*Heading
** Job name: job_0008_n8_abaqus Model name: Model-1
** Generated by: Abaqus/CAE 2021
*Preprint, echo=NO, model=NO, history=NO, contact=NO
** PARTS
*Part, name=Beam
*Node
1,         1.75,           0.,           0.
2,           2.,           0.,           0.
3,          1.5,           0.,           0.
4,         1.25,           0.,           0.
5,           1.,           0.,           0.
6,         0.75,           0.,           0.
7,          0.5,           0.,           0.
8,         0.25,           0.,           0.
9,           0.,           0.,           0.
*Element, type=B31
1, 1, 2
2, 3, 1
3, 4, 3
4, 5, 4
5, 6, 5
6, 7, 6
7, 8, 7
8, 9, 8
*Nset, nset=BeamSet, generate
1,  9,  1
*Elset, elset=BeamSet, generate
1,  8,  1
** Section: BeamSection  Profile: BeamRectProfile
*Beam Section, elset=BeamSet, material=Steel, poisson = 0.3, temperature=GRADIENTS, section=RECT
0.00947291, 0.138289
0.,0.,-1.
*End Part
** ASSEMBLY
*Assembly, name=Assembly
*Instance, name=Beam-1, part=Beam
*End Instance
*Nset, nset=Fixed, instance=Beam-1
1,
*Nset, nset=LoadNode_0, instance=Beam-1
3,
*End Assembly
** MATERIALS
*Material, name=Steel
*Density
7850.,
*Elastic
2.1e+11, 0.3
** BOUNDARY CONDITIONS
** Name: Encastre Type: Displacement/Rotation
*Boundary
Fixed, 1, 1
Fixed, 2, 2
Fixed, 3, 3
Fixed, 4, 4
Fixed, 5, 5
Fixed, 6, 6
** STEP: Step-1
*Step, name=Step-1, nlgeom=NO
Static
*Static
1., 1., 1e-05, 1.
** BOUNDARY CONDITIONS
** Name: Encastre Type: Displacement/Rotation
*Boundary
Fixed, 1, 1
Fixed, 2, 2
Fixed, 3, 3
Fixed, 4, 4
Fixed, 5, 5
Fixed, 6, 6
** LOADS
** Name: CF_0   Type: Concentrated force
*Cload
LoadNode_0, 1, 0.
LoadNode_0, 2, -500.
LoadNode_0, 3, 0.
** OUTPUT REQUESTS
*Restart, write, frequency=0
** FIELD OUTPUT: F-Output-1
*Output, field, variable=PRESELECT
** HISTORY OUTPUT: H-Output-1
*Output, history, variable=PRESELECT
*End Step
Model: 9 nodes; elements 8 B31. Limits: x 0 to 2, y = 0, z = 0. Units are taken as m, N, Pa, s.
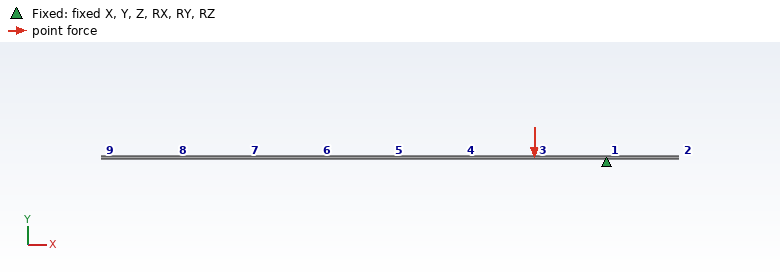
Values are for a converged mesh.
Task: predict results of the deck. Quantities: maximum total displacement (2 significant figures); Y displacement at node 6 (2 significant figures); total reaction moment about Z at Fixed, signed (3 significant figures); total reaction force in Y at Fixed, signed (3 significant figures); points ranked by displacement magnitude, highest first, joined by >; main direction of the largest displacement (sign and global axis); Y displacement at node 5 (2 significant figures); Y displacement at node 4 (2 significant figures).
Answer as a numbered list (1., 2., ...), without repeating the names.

1. 6.1e-05 m
2. -3.4e-05 m
3. -125 N·m
4. 500 N
5. node 9 > node 6 > node 5 > node 4 > node 2
6. -Y
7. -2.5e-05 m
8. -1.6e-05 m
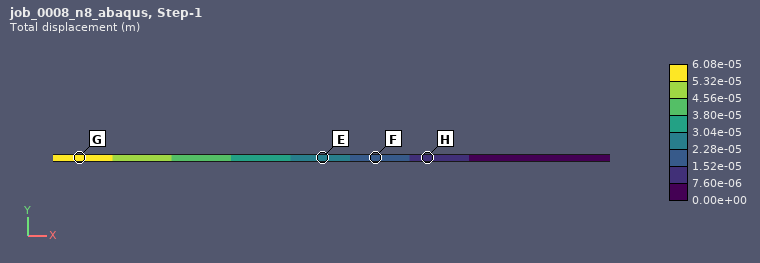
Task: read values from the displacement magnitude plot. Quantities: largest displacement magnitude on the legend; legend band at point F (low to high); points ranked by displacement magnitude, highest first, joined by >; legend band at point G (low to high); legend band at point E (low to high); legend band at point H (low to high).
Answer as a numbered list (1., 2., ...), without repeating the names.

1. 6.08e-05 m
2. 1.52e-05 to 2.28e-05 m
3. G > E > F > H
4. 5.32e-05 to 6.08e-05 m
5. 2.28e-05 to 3.04e-05 m
6. 7.60e-06 to 1.52e-05 m
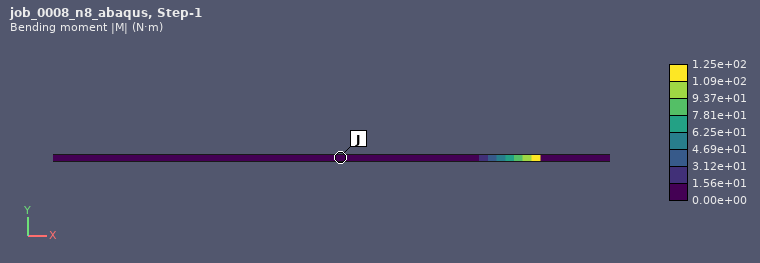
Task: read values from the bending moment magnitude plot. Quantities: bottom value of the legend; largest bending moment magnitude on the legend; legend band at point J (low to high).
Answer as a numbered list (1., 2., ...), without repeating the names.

1. 0.00e+00 N·m
2. 1.25e+02 N·m
3. 0.00e+00 to 1.56e+01 N·m
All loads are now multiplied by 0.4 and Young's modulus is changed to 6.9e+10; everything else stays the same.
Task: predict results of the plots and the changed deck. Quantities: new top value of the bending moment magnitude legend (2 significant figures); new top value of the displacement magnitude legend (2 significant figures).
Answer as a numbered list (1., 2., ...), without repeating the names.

1. 50 N·m
2. 7.4e-05 m
